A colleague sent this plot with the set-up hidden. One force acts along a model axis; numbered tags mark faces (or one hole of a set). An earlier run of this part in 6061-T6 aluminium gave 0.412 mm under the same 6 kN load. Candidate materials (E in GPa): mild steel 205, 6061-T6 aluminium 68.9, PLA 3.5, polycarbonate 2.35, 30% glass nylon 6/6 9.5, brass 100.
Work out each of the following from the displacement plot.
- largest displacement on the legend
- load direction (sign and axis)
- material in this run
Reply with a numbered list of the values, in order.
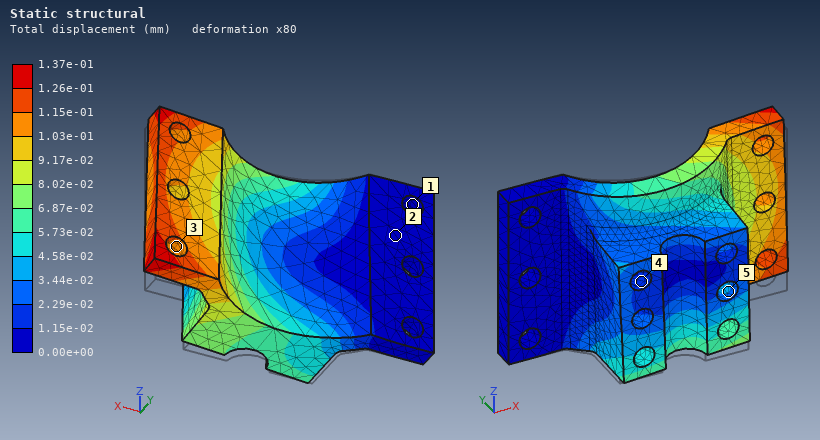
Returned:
1. 1.37e-01 mm
2. +Z
3. mild steel
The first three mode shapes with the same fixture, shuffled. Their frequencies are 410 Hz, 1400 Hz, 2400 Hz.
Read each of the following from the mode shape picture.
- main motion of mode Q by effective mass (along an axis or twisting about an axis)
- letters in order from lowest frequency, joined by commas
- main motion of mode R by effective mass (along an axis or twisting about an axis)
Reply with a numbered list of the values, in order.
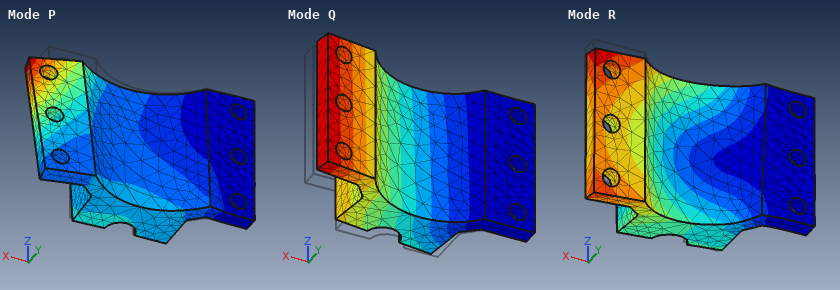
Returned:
1. along Y
2. Q, R, P
3. along Z
